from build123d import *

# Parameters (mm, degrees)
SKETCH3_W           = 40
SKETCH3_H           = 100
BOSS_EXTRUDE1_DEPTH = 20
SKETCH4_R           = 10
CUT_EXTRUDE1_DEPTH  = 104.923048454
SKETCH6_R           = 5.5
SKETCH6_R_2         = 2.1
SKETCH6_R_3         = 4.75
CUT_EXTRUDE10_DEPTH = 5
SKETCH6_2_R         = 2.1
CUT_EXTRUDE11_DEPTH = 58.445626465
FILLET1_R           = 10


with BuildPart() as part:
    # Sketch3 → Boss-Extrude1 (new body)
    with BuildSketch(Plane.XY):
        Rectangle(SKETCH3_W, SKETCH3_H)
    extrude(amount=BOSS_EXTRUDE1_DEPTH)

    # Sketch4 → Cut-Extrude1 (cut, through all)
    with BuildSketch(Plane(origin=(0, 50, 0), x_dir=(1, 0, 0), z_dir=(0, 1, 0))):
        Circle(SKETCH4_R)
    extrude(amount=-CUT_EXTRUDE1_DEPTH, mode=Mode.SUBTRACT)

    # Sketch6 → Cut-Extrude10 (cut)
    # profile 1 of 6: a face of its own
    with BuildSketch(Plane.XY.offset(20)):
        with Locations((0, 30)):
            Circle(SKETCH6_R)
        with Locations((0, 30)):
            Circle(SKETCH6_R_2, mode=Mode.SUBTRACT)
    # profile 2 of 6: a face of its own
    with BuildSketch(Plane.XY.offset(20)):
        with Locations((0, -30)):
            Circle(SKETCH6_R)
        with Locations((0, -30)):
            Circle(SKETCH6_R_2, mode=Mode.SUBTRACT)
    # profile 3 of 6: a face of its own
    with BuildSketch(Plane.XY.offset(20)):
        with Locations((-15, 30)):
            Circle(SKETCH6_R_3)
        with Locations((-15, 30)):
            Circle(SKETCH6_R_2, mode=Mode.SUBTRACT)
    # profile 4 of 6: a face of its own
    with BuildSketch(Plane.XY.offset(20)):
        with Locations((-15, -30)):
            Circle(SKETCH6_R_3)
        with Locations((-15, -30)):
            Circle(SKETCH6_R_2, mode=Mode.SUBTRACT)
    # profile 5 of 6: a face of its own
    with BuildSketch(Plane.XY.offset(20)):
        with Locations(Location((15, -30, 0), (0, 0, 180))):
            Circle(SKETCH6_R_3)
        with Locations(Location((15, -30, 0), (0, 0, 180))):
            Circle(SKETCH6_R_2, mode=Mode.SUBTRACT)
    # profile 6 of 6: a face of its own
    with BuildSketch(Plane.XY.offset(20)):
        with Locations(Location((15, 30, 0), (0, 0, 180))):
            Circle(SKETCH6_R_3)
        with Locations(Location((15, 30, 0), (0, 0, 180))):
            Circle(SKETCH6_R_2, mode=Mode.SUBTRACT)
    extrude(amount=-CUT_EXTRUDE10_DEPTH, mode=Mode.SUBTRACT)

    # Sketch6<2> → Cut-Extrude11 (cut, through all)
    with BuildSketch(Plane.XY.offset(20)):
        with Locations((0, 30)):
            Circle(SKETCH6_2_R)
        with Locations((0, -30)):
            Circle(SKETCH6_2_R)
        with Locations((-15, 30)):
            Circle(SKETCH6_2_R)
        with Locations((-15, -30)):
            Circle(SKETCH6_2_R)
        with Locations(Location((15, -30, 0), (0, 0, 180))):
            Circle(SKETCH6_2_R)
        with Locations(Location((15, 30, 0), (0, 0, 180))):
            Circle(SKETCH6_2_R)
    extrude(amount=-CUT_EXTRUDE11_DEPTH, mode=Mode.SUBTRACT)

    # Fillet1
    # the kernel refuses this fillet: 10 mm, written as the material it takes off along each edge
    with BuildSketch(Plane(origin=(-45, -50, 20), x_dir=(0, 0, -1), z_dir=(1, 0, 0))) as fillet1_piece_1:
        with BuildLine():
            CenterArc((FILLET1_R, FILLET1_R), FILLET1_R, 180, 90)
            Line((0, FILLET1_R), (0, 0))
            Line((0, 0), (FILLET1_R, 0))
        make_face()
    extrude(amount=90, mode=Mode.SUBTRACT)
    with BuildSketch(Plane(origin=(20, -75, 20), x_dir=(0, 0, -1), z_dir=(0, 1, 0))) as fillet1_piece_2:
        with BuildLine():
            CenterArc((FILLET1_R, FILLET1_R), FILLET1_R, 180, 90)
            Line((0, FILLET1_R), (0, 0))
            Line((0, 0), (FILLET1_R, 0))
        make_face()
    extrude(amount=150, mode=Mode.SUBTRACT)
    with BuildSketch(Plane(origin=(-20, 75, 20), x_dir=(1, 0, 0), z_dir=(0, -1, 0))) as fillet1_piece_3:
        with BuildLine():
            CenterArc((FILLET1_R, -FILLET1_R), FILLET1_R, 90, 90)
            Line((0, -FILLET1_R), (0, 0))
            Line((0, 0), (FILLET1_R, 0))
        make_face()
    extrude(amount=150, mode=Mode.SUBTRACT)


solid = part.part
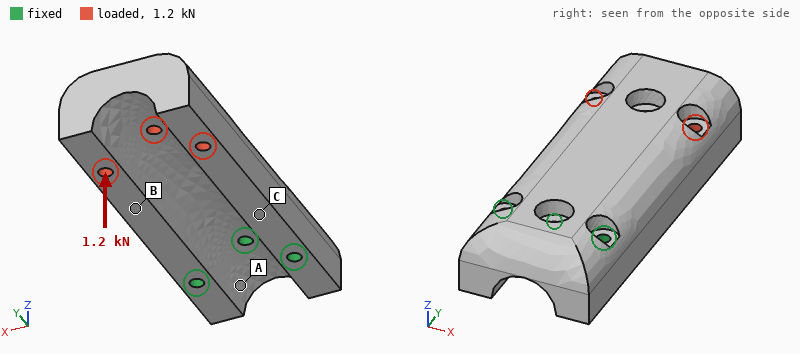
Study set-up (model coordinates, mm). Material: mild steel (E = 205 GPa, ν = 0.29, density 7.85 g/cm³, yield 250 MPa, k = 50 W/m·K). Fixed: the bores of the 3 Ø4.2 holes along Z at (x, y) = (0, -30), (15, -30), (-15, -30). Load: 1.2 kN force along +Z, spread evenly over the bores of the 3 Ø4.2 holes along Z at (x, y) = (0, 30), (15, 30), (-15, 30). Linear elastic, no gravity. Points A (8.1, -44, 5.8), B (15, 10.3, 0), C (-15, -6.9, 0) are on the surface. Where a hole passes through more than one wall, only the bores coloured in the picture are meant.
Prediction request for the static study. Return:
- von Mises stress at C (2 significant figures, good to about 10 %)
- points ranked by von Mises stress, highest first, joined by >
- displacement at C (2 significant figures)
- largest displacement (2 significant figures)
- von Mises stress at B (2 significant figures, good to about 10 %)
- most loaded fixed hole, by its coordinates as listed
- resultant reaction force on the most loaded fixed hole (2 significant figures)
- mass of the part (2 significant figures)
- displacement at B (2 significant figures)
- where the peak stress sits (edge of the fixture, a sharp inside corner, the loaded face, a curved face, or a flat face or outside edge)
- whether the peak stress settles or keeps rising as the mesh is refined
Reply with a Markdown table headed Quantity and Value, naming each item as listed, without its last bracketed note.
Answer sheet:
| Quantity | Value |
|---|---|
| von Mises stress at C | 29 MPa |
| points ranked by von Mises stress, highest first, joined by > | C > B > A |
| displacement at C | 9.6 µm |
| largest displacement | 49 µm |
| von Mises stress at B | 15 MPa |
| most loaded fixed hole, by its coordinates as listed | (0, -30) |
| resultant reaction force on the most loaded fixed hole | 2.0 kN |
| mass of the part | 440 g |
| displacement at B | 20 µm |
| where the peak stress sits | edge of the fixture |
| whether the peak stress settles or keeps rising as the mesh is refined | keeps rising |
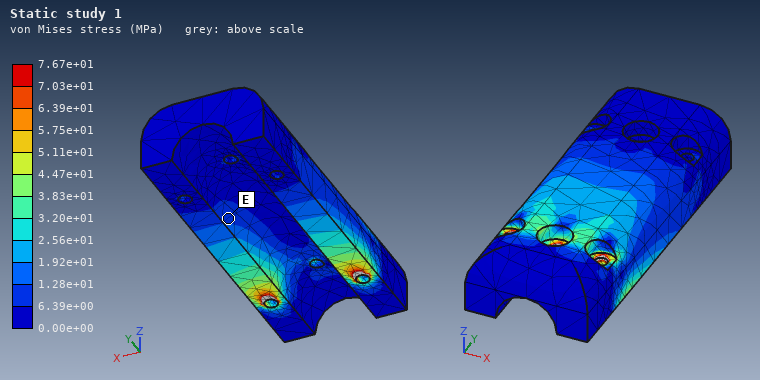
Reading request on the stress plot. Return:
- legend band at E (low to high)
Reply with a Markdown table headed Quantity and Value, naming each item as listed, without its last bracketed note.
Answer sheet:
| Quantity | Value |
|---|---|
| legend band at E | 6.39e+00 to 1.28e+01 MPa |
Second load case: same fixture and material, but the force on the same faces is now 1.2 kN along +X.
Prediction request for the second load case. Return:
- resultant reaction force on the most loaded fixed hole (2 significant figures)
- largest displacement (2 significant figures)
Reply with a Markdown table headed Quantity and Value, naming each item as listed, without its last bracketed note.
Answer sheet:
| Quantity | Value |
|---|---|
| resultant reaction force on the most loaded fixed hole | 2.3 kN |
| largest displacement | 16 µm |
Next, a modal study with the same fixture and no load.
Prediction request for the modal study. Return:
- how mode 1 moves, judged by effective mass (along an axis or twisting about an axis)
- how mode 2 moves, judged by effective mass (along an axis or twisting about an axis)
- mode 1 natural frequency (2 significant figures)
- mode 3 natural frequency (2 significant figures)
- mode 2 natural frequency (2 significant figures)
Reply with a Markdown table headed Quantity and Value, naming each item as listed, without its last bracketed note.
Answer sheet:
| Quantity | Value |
|---|---|
| how mode 1 moves, judged by effective mass | along Z |
| how mode 2 moves, judged by effective mass | along X |
| mode 1 natural frequency | 2100 Hz |
| mode 3 natural frequency | 6100 Hz |
| mode 2 natural frequency | 3900 Hz |
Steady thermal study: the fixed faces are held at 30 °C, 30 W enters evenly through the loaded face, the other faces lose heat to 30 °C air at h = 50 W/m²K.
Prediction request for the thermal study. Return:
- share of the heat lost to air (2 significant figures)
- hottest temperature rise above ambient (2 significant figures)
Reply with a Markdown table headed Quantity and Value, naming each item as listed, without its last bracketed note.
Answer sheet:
| Quantity | Value |
|---|---|
| share of the heat lost to air | 45 % |
| hottest temperature rise above ambient | 43 K |
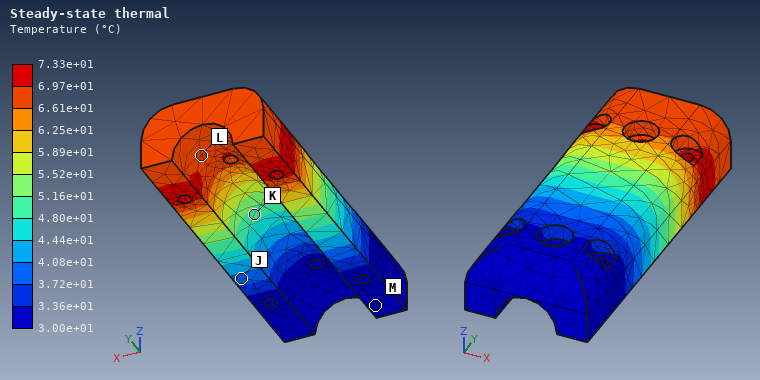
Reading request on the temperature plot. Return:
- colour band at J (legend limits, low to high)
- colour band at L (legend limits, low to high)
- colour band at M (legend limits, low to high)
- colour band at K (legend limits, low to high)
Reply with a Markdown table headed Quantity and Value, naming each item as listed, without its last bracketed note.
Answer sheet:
| Quantity | Value |
|---|---|
| colour band at J | 3.72e+01 to 4.08e+01 °C |
| colour band at L | 6.61e+01 to 6.97e+01 °C |
| colour band at M | 3.00e+01 to 3.36e+01 °C |
| colour band at K | 4.80e+01 to 5.16e+01 °C |
